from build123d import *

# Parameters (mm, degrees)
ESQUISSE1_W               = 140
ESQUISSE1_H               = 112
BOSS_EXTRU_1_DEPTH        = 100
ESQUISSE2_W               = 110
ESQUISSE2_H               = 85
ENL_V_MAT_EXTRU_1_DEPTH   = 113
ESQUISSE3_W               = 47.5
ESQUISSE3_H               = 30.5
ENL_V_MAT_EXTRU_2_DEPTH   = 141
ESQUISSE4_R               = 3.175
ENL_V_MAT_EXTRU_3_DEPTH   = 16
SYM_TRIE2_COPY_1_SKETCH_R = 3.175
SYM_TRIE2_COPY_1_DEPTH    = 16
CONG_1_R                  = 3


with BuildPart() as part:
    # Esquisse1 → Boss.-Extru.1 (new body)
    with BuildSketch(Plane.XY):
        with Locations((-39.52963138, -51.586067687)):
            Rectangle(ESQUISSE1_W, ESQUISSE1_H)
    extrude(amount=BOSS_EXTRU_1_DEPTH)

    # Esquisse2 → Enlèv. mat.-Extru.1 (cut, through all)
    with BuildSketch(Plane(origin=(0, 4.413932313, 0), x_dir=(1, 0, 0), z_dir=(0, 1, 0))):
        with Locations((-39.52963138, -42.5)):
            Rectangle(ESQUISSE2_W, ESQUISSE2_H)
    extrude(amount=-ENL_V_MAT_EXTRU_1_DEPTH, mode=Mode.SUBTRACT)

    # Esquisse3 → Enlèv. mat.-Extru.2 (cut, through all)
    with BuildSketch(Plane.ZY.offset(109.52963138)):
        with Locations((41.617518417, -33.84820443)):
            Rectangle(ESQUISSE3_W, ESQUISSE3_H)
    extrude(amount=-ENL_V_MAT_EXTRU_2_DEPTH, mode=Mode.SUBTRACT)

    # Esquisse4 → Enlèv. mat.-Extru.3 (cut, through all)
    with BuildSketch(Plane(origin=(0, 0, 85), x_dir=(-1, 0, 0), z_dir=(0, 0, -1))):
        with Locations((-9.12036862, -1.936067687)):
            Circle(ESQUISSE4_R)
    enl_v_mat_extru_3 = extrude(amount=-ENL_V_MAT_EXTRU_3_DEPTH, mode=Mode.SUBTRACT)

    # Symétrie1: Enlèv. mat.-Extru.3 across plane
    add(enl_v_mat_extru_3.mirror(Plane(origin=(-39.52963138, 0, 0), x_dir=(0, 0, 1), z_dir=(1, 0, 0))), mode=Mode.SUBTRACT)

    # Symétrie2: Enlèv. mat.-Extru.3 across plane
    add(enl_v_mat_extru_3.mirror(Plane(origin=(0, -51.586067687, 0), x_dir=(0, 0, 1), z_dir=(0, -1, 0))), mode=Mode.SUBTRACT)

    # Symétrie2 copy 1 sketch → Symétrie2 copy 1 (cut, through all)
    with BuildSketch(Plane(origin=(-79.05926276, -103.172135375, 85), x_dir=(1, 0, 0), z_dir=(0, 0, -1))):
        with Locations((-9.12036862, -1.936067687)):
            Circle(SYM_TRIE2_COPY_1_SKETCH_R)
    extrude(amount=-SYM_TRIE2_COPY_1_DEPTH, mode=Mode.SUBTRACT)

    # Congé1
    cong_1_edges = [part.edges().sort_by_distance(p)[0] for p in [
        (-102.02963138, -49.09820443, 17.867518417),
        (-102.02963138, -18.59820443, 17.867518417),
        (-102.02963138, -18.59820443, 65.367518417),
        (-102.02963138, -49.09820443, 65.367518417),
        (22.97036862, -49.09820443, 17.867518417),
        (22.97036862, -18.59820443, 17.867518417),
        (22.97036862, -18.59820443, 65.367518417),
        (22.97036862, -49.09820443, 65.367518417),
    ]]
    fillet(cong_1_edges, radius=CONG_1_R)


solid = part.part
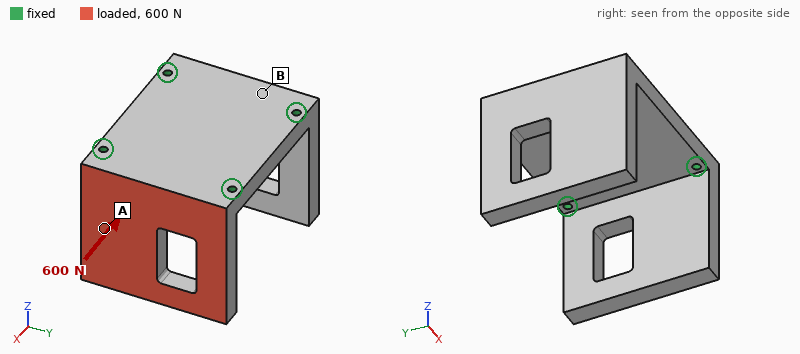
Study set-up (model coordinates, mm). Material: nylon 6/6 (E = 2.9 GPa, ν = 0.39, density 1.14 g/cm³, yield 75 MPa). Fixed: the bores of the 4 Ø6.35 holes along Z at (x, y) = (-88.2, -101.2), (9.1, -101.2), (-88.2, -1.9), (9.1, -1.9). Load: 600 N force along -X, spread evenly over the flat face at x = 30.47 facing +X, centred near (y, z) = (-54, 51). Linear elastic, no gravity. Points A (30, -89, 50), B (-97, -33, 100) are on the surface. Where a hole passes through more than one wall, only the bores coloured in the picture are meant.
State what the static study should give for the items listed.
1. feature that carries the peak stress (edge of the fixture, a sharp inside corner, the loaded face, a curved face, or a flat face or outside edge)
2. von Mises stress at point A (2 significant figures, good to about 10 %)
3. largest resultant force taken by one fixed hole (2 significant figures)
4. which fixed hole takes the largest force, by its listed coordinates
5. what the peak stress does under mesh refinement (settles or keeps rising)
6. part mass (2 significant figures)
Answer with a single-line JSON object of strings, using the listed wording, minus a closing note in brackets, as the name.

{"feature that carries the peak stress": "edge of the fixture", "von Mises stress at point A": "2.3 MPa", "largest resultant force taken by one fixed hole": "220 N", "which fixed hole takes the largest force, by its listed coordinates": "(9.1, -101.2)", "what the peak stress does under mesh refinement": "keeps rising", "part mass": "540 g"}
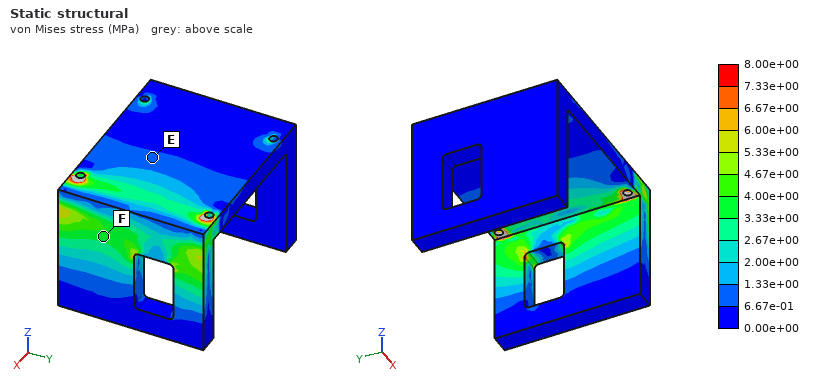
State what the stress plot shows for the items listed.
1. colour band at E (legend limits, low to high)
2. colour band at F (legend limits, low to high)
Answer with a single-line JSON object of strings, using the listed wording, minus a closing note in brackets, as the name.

{"colour band at E": "6.67e-01 to 1.33e+00 MPa", "colour band at F": "3.33e+00 to 4.00e+00 MPa"}
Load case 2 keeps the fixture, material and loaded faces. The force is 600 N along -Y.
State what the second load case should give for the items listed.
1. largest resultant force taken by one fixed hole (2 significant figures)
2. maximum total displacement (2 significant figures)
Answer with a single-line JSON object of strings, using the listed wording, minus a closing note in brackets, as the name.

{"largest resultant force taken by one fixed hole": "410 N", "maximum total displacement": "0.10 mm"}
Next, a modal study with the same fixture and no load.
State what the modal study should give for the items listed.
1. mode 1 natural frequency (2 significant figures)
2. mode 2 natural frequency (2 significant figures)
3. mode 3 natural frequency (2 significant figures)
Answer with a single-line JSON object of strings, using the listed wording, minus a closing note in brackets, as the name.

{"mode 1 natural frequency": "350 Hz", "mode 2 natural frequency": "360 Hz", "mode 3 natural frequency": "740 Hz"}
